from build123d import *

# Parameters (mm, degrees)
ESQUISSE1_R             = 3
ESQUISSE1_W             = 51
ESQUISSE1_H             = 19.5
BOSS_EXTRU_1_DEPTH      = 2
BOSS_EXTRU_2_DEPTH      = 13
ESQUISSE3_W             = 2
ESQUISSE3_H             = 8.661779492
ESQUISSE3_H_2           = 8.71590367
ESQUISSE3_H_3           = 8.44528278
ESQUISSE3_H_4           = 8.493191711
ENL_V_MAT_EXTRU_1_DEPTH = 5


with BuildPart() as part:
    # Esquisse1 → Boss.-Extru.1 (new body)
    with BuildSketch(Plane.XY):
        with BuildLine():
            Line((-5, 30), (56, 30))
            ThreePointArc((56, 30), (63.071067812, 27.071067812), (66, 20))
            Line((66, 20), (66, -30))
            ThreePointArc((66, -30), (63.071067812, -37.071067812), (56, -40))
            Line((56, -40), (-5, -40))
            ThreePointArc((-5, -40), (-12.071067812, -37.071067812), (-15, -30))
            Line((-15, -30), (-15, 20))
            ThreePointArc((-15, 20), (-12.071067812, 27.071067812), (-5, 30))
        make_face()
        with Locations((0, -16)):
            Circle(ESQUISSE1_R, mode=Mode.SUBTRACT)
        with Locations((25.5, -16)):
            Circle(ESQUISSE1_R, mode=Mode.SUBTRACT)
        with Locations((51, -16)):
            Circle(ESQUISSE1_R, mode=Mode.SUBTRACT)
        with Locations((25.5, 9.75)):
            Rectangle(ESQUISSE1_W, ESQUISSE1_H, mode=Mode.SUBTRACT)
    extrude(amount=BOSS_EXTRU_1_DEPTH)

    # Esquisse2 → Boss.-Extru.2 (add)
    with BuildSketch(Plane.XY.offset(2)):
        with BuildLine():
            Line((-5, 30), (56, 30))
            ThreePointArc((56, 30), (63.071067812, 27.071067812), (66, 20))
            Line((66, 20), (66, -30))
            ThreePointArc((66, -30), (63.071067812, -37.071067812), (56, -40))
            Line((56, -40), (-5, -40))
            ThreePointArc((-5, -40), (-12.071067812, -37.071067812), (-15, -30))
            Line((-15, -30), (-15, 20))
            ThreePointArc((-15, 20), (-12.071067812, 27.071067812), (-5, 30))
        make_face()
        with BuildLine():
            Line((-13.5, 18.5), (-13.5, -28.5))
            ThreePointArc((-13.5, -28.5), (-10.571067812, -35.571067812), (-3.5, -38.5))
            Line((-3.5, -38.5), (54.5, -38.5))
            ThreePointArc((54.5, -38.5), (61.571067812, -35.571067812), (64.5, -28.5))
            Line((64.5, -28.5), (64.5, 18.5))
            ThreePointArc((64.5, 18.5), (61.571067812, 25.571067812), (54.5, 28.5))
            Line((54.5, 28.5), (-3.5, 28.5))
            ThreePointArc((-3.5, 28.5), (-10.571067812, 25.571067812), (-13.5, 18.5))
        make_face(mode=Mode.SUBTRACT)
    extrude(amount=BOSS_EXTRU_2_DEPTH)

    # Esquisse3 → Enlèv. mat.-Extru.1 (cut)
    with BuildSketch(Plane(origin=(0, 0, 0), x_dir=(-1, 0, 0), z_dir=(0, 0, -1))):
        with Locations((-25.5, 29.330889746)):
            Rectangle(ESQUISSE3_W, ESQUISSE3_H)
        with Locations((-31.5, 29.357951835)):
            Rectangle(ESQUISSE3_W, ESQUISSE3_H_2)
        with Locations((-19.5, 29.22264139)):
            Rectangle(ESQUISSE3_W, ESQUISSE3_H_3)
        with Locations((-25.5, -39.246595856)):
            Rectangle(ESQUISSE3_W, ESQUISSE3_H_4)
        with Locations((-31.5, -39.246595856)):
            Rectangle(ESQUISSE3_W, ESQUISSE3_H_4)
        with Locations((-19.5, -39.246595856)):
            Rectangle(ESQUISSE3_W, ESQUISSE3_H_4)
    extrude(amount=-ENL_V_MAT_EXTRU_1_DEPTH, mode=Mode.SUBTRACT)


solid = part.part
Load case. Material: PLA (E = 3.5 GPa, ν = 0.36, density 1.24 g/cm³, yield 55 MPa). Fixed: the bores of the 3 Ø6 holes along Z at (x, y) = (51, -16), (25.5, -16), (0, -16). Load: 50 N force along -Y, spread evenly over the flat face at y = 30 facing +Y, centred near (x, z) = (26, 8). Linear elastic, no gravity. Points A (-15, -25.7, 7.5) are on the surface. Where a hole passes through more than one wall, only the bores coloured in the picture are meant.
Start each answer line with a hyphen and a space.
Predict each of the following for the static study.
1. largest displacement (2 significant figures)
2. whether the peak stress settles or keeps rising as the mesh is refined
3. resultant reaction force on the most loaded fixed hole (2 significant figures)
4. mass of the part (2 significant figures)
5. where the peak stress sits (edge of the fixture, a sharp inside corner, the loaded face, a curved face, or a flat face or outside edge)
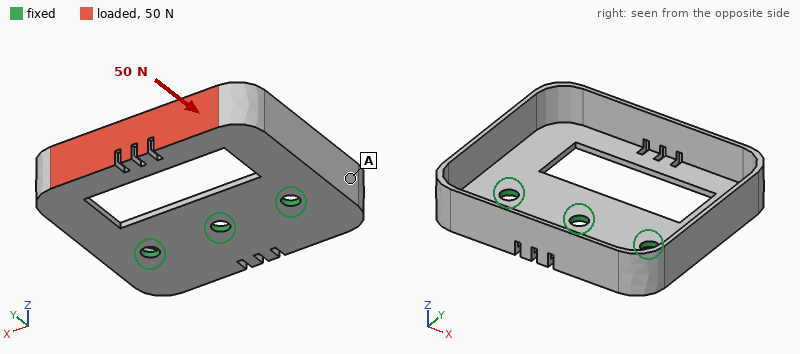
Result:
- 1.2 mm
- keeps rising
- 35 N
- 18 g
- a sharp inside corner
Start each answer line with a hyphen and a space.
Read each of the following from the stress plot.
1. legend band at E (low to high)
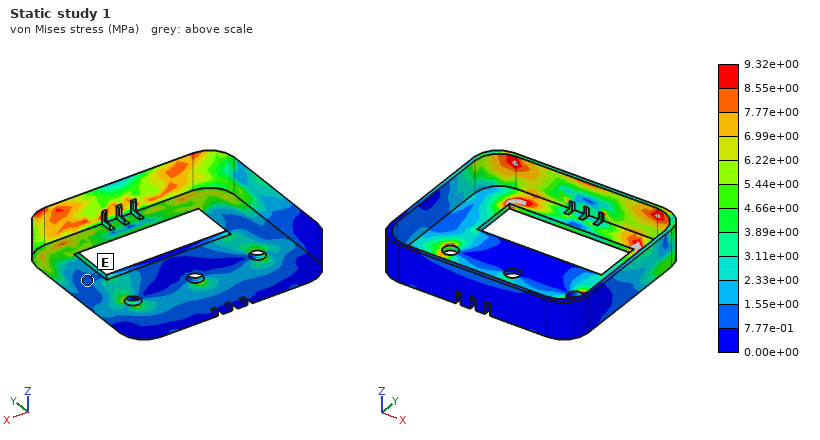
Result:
- 7.77e-01 to 1.55e+00 MPa
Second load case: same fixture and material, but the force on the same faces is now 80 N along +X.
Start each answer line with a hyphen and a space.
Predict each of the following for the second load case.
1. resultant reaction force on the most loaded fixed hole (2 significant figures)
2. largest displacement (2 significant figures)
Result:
- 64 N
- 1.1 mm
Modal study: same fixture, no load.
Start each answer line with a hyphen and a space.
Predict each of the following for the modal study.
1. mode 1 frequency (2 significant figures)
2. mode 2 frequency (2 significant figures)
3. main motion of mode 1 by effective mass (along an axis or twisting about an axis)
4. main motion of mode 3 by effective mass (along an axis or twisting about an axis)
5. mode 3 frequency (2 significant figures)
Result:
- 290 Hz
- 360 Hz
- along Z
- along Z
- 990 Hz
